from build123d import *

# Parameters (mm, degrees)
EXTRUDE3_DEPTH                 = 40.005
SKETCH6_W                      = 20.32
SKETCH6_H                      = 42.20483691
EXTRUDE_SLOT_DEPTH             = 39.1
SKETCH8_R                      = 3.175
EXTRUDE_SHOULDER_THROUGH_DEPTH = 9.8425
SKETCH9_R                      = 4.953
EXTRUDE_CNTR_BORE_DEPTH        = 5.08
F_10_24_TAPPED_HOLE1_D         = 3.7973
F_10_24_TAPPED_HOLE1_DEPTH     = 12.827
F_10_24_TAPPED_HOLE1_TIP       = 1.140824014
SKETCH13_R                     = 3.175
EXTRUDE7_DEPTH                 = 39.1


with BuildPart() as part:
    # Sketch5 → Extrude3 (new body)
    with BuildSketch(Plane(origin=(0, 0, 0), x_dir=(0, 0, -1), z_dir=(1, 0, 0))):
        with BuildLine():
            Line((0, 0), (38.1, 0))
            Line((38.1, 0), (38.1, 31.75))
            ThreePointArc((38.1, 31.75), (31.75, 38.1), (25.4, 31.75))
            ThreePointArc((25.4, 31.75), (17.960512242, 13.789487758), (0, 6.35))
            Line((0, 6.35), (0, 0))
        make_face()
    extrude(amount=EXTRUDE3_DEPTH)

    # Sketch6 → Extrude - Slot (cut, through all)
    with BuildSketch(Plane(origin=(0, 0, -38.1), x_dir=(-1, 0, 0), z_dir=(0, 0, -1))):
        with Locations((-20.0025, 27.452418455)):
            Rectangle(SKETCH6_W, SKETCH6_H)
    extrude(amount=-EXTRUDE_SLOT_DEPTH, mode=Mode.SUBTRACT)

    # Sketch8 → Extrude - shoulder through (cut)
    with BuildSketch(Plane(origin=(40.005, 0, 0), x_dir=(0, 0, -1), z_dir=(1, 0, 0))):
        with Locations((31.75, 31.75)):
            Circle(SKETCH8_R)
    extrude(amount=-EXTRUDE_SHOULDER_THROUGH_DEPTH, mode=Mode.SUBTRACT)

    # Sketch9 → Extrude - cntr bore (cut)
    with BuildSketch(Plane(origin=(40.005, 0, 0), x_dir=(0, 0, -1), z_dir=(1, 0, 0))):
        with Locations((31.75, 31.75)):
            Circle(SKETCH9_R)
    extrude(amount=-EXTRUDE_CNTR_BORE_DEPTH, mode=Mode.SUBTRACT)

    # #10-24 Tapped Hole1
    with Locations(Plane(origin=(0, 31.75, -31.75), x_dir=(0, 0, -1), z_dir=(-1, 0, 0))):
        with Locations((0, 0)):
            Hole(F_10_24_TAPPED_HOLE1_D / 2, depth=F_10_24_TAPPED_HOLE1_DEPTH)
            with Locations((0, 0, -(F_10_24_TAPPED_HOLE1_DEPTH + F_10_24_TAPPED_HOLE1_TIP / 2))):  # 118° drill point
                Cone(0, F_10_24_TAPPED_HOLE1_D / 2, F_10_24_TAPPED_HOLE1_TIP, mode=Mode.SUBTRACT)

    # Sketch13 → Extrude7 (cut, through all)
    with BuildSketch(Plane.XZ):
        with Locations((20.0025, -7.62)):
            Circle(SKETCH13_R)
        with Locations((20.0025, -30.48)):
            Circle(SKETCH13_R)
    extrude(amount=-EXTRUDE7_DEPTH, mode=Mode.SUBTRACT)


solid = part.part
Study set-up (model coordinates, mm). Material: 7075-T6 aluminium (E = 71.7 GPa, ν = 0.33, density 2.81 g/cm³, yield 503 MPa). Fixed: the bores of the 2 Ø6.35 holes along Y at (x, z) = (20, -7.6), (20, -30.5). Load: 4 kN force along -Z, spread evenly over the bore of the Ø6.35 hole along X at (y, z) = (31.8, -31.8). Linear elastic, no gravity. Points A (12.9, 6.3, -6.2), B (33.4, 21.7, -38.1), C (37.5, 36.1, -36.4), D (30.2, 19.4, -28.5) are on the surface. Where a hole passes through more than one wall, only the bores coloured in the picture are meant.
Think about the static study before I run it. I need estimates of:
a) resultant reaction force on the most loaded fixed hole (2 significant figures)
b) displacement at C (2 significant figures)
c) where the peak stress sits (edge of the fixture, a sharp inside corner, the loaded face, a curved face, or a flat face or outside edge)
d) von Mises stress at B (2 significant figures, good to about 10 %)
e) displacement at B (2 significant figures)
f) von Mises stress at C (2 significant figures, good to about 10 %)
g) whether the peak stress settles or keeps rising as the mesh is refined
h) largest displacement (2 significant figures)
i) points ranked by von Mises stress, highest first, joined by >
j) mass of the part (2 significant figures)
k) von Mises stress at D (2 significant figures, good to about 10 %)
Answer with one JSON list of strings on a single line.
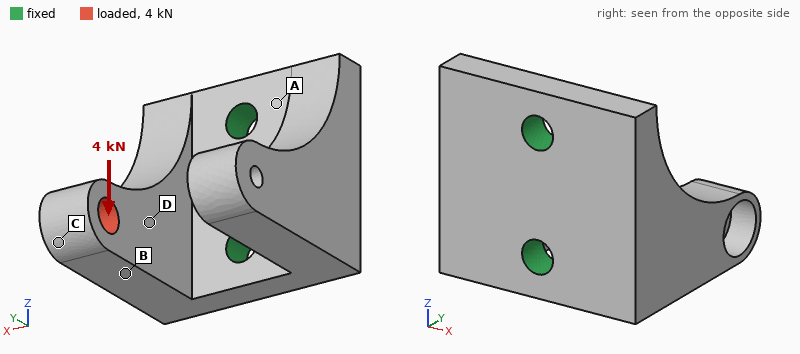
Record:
["5.1 kN", "0.39 mm", "edge of the fixture", "140 MPa", "0.22 mm", "72 MPa", "keeps rising", "0.42 mm", "B > D > C > A", "53 g", "100 MPa"]
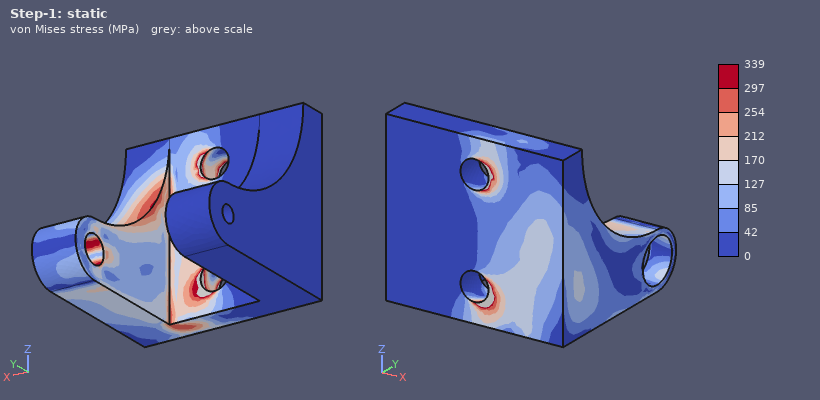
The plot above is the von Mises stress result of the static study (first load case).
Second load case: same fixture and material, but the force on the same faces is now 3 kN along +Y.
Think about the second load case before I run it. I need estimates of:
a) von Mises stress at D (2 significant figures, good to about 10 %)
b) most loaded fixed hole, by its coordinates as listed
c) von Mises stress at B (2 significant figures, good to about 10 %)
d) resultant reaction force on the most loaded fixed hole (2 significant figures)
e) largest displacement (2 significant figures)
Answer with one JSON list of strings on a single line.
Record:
["48 MPa", "(20, -30.5)", "47 MPa", "2.9 kN", "0.14 mm"]
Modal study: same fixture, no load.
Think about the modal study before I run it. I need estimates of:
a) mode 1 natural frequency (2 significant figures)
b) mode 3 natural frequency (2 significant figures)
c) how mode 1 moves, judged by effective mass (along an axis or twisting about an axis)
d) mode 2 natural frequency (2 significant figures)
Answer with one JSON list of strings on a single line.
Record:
["4000 Hz", "7800 Hz", "along X", "4500 Hz"]
